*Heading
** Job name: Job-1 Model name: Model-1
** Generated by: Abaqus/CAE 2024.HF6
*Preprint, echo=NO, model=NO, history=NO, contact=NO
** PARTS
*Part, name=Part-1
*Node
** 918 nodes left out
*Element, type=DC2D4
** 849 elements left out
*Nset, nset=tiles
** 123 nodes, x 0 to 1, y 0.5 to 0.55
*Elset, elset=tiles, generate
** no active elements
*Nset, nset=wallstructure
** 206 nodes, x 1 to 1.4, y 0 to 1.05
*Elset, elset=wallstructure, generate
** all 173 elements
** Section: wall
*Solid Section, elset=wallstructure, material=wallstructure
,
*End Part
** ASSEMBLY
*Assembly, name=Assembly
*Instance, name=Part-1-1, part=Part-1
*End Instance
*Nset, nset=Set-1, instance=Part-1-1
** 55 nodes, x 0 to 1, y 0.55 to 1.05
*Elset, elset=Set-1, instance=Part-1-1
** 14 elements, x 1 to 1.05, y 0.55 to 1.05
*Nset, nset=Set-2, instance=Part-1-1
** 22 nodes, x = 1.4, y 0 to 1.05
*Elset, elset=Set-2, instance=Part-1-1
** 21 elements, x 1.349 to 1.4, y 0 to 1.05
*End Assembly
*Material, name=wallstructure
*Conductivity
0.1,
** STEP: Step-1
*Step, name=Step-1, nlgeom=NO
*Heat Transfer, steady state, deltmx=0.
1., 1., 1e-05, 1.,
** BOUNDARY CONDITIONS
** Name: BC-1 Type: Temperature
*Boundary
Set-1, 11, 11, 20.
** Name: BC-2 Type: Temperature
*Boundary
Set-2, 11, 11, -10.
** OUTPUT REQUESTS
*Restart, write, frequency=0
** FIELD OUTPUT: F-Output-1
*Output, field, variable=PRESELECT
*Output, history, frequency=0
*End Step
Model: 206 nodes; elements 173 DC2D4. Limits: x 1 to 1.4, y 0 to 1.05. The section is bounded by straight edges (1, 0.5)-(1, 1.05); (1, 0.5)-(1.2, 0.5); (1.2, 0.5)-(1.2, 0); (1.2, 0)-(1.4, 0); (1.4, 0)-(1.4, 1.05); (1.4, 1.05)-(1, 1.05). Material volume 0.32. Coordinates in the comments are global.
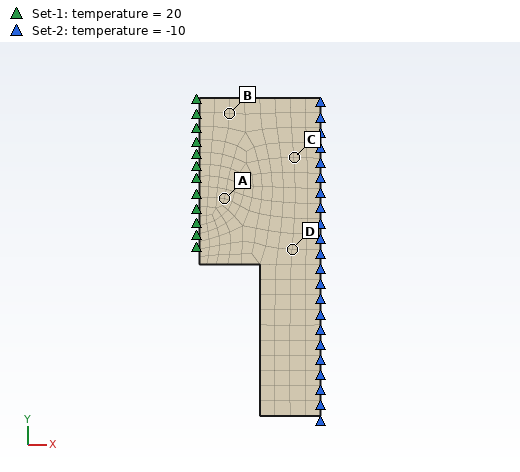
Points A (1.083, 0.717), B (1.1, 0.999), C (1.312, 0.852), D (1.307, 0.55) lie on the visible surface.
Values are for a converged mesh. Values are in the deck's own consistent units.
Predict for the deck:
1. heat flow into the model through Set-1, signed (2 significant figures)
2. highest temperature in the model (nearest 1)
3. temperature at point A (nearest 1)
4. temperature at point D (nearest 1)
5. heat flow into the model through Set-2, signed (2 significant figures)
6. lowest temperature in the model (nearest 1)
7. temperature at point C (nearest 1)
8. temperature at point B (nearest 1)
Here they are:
4.3
20
13
-5
-4.3
-10
-4
12
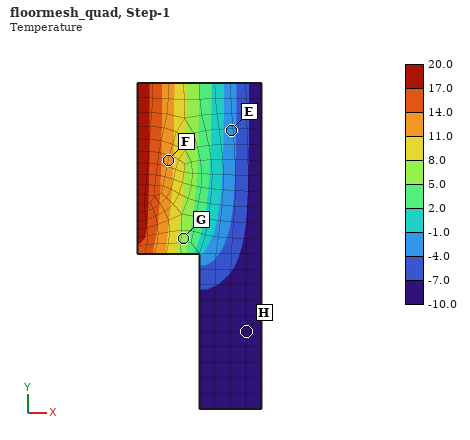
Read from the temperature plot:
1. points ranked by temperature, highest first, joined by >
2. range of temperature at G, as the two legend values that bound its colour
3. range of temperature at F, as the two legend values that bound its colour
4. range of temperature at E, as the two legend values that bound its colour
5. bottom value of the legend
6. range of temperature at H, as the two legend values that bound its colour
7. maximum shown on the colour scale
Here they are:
F > G > E > H
5.0 to 8.0
11.0 to 14.0
-4.0 to -1.0
-10.0
-10.0 to -7.0
20.0
